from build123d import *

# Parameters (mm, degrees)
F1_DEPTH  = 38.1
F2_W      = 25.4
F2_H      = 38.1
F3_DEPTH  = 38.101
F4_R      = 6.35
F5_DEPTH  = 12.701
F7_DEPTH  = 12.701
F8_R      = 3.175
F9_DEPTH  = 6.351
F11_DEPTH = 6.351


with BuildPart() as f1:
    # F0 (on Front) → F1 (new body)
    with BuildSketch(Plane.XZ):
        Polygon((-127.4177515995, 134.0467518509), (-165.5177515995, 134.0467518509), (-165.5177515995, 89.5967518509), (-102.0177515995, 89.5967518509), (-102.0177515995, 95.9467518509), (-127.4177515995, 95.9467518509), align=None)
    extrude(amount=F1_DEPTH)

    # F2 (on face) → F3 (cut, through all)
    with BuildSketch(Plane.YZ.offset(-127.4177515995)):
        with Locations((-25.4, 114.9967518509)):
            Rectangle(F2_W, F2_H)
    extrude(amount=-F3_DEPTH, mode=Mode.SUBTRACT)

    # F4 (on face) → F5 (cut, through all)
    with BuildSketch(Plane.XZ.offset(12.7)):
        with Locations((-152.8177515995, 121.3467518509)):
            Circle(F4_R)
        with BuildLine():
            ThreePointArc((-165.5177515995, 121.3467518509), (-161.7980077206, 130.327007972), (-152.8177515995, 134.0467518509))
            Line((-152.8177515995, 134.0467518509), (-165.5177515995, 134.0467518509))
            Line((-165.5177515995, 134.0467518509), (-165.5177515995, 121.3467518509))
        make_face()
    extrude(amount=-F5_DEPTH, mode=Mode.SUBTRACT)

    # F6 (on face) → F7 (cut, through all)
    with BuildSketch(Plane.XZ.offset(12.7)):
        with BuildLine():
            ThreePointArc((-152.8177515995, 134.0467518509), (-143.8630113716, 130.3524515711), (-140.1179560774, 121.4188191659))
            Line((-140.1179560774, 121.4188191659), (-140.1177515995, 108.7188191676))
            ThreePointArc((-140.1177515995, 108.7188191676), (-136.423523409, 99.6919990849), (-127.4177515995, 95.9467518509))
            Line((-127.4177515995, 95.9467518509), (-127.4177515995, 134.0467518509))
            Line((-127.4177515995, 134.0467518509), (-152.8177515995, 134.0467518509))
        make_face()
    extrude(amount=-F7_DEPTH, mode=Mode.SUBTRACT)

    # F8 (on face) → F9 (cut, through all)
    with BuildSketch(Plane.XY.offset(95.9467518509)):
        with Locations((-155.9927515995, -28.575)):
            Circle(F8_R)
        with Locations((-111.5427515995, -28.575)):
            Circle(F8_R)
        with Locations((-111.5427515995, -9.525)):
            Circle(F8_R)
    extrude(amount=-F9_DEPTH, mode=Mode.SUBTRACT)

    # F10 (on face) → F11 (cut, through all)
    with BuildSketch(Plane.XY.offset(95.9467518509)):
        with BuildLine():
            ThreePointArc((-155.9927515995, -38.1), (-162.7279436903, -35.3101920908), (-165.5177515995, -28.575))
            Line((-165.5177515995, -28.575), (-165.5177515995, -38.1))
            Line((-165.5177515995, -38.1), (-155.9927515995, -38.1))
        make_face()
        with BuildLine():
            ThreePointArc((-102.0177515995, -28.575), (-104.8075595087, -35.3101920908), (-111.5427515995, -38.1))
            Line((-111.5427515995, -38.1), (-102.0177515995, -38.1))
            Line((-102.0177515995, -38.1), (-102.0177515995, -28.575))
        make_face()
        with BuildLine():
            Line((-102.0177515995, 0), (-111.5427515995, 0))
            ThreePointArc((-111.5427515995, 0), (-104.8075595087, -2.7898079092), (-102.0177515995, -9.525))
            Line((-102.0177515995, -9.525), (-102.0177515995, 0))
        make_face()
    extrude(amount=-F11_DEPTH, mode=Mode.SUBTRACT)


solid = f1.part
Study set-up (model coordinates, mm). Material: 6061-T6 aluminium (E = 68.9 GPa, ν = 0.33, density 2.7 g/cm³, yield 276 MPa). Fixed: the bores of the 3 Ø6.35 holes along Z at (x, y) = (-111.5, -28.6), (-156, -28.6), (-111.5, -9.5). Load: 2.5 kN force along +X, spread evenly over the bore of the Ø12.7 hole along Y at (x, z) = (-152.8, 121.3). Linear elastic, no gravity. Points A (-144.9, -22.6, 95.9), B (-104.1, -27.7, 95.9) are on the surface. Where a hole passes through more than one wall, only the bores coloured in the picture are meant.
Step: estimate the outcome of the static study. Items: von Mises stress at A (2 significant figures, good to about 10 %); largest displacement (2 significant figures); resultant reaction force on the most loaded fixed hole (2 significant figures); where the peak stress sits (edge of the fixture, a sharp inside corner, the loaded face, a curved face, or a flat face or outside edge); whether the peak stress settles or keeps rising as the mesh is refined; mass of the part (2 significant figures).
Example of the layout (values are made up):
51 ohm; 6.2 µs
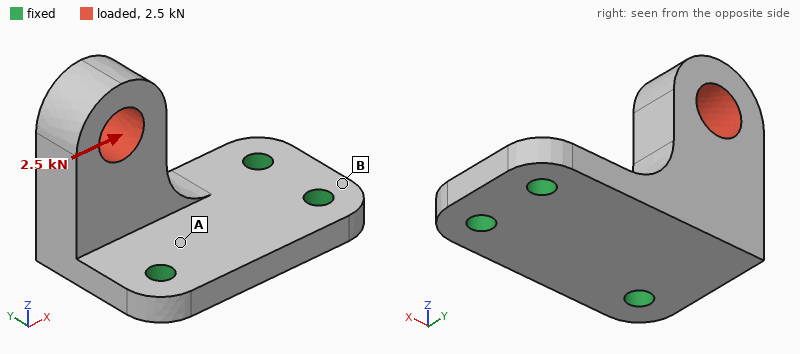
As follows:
56 MPa; 0.28 mm; 1.9 kN; edge of the fixture; keeps rising; 67 g
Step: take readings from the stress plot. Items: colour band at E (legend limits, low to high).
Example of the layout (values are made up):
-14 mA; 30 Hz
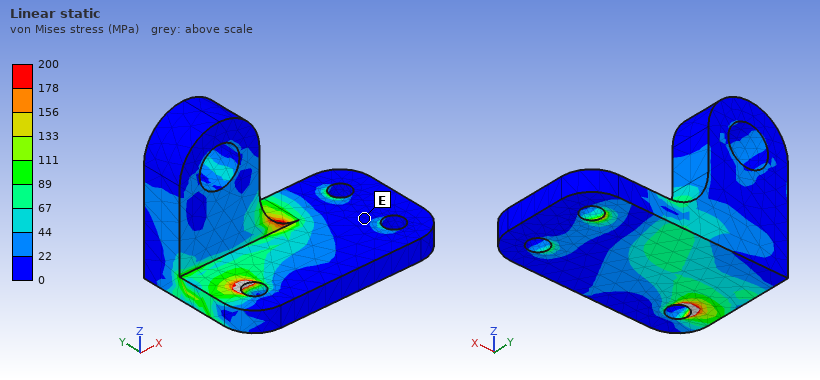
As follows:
0 to 22 MPa
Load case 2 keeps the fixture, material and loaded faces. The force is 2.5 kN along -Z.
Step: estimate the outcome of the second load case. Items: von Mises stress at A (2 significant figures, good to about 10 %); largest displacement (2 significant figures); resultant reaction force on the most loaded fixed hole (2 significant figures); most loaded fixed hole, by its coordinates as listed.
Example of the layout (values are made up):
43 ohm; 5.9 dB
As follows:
61 MPa; 0.31 mm; 2.0 kN; (-156, -28.6)
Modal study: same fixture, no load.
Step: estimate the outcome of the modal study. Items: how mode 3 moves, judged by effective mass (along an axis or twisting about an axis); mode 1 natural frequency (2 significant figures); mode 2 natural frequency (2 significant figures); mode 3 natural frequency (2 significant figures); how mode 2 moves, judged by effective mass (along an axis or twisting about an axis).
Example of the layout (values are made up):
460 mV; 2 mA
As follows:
along Z; 2400 Hz; 5000 Hz; 7700 Hz; along X
